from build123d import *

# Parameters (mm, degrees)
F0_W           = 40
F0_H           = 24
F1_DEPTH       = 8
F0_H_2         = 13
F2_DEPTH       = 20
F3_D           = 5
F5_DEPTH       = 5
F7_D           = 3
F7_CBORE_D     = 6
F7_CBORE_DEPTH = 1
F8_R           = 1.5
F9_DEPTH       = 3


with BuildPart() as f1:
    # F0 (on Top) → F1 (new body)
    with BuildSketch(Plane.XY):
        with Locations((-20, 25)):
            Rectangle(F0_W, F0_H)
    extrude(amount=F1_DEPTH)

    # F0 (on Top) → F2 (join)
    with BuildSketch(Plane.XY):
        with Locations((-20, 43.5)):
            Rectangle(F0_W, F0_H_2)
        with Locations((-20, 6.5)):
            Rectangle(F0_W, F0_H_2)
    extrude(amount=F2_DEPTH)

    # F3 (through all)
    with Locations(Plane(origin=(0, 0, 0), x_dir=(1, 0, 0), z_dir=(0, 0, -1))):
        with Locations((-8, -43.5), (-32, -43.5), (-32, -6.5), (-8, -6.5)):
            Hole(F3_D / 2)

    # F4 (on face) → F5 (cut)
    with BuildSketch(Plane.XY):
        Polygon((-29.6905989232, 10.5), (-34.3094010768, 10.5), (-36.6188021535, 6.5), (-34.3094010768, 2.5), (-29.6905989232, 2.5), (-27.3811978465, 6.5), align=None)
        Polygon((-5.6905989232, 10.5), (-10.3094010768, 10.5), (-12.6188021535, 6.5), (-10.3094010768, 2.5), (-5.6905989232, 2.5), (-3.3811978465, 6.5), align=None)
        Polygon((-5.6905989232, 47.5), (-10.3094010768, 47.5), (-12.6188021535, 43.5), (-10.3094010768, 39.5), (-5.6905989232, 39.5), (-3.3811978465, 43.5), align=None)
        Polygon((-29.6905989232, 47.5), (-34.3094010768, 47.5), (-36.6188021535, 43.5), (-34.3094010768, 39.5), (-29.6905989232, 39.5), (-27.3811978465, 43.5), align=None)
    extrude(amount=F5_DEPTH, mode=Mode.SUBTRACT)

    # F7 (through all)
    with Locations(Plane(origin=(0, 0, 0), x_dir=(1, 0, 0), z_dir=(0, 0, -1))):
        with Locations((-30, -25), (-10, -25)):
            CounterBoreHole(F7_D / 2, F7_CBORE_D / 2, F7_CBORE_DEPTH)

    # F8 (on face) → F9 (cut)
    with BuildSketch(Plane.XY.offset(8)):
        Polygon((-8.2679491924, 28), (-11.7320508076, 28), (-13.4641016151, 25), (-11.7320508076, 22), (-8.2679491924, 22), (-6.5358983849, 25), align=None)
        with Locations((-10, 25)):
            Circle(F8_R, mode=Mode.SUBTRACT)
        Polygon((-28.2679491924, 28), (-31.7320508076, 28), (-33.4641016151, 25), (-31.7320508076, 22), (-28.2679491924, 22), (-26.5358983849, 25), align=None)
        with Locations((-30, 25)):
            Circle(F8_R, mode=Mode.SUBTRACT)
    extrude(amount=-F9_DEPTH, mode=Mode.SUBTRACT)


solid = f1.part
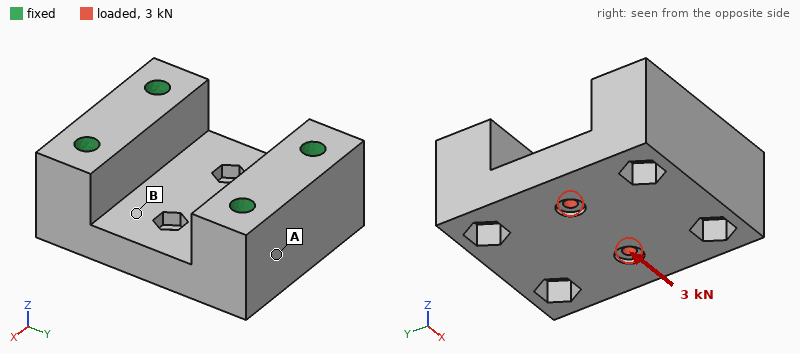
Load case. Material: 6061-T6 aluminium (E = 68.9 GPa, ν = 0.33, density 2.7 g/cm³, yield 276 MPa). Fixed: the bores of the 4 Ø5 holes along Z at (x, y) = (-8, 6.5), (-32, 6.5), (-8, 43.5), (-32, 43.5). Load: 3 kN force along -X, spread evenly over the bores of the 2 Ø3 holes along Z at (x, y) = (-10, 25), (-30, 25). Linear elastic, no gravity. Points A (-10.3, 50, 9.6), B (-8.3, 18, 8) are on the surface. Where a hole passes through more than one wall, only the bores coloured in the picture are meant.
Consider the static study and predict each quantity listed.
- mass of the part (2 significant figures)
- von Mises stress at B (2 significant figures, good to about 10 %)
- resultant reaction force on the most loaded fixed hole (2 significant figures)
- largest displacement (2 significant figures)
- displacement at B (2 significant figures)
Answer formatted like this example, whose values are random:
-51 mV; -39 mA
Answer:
70 g; 7.8 MPa; 910 N; 5.9 µm; 2.6 µm
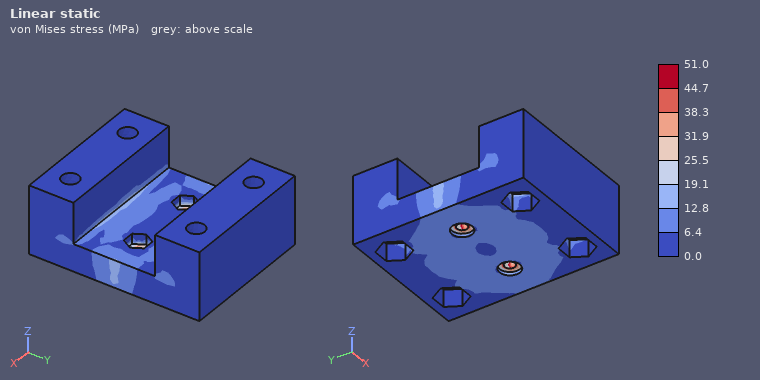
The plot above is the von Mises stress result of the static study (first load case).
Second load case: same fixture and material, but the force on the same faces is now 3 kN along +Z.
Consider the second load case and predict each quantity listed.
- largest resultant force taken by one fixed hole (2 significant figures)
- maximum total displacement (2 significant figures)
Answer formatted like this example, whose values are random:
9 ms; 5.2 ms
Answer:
1.0 kN; 13 µm
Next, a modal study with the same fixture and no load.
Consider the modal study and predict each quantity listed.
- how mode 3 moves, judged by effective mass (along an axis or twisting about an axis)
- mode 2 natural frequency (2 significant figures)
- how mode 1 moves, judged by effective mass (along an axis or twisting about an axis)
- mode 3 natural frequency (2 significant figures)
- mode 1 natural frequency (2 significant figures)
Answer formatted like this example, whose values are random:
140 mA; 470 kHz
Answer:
along X; 31 kHz; along Z; 36 kHz; 28 kHz
